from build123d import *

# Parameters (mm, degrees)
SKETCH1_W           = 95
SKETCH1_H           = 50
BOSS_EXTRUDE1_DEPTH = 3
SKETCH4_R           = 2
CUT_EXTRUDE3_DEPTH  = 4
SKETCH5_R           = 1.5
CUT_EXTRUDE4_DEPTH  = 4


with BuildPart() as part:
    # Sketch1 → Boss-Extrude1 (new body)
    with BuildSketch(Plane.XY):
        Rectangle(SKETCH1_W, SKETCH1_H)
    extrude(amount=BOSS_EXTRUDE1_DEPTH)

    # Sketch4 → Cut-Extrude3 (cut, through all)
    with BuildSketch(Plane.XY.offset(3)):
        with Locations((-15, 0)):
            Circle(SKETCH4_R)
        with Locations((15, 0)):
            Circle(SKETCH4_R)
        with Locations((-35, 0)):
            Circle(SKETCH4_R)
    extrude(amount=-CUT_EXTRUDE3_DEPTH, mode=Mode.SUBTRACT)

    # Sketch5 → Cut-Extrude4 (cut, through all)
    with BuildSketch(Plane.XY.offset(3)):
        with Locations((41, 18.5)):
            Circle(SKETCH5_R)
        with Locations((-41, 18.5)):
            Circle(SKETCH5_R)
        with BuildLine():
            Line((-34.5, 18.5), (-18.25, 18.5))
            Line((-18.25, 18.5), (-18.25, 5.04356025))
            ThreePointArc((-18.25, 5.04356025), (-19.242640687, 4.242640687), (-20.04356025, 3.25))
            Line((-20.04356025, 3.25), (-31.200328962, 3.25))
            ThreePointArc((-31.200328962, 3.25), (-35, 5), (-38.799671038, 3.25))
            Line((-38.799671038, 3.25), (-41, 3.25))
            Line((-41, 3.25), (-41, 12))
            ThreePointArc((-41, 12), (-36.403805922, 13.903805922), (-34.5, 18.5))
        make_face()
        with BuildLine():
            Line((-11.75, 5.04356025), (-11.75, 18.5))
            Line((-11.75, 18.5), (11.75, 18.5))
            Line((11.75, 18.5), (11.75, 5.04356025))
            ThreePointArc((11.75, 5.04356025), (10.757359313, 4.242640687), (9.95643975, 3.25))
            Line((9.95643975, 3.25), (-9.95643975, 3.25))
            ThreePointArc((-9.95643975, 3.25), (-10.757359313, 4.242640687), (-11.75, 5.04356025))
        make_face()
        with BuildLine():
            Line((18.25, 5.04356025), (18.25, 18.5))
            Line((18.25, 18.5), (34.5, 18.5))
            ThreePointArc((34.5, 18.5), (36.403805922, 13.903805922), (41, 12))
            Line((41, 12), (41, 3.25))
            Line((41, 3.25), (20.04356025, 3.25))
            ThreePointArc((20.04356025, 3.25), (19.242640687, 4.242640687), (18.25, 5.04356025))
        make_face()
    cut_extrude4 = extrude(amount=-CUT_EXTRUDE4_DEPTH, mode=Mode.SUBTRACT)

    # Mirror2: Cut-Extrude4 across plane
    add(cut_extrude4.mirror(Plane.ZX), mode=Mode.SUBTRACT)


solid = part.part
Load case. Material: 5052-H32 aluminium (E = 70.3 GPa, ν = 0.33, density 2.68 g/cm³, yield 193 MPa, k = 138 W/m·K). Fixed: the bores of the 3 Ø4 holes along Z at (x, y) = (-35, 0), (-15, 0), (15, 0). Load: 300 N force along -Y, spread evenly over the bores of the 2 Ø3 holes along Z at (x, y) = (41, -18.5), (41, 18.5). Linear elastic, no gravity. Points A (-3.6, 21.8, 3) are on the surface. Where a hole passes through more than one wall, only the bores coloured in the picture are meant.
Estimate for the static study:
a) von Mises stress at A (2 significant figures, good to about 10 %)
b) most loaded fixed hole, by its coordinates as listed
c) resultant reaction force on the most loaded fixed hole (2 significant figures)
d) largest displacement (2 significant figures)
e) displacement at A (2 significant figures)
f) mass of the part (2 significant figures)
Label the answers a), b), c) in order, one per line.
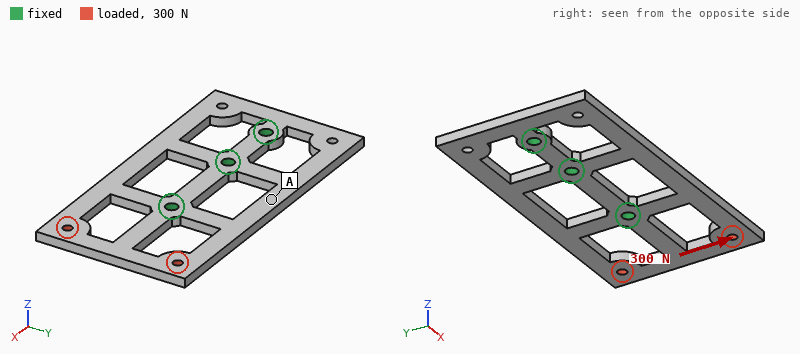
a) 7.6 MPa
b) (15, 0)
c) 410 N
d) 59 µm
e) 13 µm
f) 22 g
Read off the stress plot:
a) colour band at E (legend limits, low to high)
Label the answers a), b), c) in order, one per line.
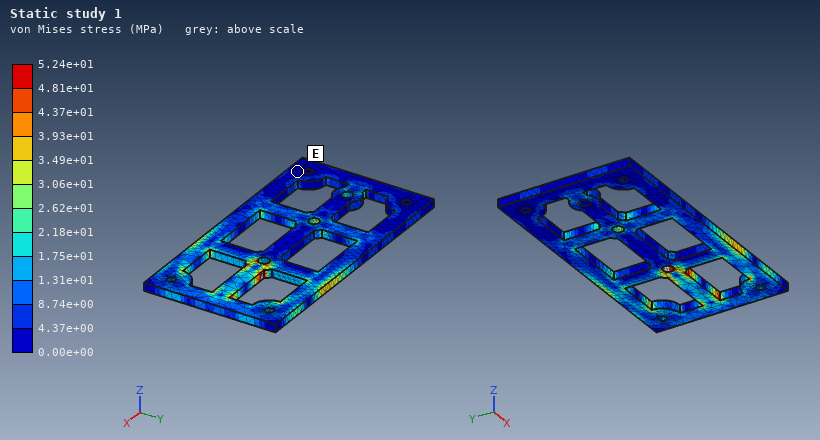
a) 0.00e+00 to 4.37e+00 MPa
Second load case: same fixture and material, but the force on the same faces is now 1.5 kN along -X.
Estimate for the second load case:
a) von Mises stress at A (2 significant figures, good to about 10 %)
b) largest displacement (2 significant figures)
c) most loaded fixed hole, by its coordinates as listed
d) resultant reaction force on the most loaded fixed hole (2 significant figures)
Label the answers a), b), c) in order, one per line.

a) 16 MPa
b) 40 µm
c) (15, 0)
d) 900 N
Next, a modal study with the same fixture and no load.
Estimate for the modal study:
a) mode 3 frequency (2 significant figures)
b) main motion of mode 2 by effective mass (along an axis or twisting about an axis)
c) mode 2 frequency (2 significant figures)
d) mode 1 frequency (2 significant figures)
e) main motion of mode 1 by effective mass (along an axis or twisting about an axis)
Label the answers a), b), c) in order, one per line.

a) 2300 Hz
b) twisting about X
c) 1800 Hz
d) 1400 Hz
e) along Z
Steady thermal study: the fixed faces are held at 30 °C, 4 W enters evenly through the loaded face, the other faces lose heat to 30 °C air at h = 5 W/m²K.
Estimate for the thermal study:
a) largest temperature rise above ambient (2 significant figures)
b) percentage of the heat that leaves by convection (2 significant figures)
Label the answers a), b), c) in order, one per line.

a) 18 K
b) 4.9 %
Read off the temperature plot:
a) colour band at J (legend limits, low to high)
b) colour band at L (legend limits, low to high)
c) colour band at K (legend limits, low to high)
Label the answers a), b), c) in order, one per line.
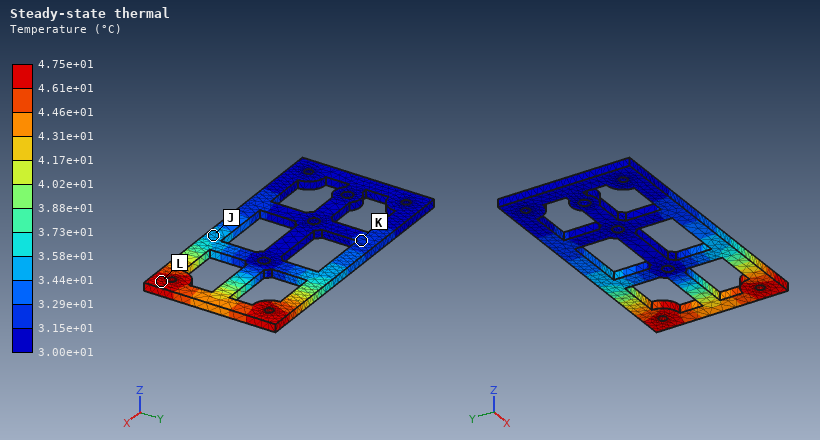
a) 3.44e+01 to 3.58e+01 °C
b) 4.61e+01 to 4.75e+01 °C
c) 3.15e+01 to 3.29e+01 °C
